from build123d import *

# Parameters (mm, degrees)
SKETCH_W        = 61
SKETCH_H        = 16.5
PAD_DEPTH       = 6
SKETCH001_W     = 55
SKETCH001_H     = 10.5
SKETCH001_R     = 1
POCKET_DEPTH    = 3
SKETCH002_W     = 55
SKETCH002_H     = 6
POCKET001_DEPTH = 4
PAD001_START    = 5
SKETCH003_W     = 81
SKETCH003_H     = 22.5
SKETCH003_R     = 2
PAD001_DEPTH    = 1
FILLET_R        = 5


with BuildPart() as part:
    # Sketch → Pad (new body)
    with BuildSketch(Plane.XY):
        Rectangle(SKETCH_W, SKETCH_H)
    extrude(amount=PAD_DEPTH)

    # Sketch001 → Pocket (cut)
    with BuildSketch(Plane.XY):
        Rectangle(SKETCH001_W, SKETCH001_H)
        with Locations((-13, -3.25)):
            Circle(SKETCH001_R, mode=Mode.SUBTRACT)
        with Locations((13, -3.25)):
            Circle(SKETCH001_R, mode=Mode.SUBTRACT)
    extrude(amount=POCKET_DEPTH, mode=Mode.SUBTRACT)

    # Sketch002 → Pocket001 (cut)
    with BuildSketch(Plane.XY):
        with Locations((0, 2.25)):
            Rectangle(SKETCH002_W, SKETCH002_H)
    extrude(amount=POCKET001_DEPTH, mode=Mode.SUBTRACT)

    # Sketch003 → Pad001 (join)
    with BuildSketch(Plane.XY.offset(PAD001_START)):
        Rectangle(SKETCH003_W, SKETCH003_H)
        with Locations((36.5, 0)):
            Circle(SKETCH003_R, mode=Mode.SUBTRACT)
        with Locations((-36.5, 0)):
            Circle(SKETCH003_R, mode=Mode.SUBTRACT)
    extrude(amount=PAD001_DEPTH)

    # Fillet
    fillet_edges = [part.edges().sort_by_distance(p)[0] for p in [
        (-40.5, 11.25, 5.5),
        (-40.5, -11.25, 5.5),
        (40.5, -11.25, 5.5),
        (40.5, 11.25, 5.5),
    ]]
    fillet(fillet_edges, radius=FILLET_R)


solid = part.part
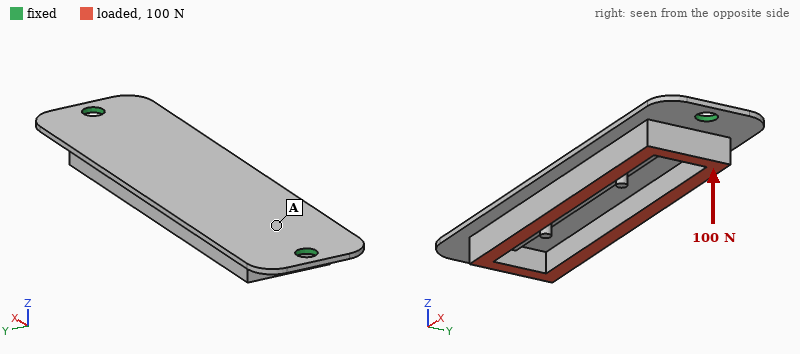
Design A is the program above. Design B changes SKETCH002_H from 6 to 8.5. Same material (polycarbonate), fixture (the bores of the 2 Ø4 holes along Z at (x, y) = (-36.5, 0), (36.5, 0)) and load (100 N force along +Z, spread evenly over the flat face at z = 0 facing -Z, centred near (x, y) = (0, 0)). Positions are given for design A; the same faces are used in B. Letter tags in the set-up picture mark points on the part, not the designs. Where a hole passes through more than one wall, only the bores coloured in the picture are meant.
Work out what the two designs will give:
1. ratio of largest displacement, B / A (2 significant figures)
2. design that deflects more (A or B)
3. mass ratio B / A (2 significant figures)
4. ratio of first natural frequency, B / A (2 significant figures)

1.5
B
0.93
1.0
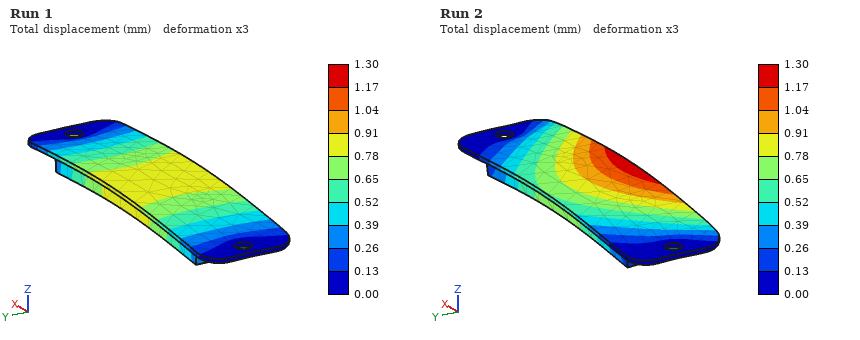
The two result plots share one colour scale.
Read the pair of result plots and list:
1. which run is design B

Run 2
